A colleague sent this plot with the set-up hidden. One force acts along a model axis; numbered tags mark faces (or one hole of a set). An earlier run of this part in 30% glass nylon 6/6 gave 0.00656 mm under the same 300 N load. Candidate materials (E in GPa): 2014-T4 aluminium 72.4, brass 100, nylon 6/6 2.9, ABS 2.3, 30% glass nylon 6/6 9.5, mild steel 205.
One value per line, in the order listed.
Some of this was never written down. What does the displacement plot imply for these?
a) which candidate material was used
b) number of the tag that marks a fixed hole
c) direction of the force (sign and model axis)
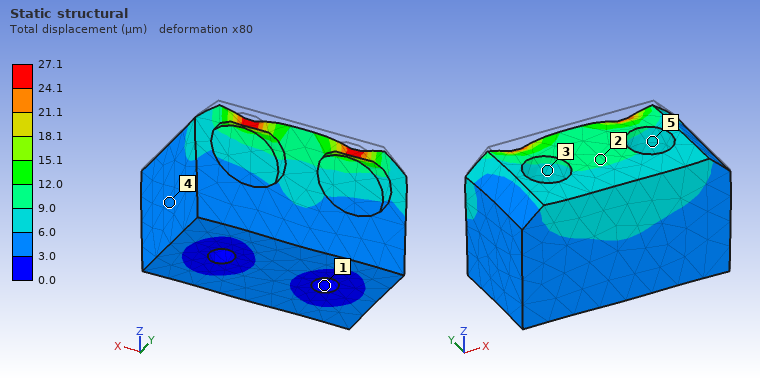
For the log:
ABS
1
-Z
